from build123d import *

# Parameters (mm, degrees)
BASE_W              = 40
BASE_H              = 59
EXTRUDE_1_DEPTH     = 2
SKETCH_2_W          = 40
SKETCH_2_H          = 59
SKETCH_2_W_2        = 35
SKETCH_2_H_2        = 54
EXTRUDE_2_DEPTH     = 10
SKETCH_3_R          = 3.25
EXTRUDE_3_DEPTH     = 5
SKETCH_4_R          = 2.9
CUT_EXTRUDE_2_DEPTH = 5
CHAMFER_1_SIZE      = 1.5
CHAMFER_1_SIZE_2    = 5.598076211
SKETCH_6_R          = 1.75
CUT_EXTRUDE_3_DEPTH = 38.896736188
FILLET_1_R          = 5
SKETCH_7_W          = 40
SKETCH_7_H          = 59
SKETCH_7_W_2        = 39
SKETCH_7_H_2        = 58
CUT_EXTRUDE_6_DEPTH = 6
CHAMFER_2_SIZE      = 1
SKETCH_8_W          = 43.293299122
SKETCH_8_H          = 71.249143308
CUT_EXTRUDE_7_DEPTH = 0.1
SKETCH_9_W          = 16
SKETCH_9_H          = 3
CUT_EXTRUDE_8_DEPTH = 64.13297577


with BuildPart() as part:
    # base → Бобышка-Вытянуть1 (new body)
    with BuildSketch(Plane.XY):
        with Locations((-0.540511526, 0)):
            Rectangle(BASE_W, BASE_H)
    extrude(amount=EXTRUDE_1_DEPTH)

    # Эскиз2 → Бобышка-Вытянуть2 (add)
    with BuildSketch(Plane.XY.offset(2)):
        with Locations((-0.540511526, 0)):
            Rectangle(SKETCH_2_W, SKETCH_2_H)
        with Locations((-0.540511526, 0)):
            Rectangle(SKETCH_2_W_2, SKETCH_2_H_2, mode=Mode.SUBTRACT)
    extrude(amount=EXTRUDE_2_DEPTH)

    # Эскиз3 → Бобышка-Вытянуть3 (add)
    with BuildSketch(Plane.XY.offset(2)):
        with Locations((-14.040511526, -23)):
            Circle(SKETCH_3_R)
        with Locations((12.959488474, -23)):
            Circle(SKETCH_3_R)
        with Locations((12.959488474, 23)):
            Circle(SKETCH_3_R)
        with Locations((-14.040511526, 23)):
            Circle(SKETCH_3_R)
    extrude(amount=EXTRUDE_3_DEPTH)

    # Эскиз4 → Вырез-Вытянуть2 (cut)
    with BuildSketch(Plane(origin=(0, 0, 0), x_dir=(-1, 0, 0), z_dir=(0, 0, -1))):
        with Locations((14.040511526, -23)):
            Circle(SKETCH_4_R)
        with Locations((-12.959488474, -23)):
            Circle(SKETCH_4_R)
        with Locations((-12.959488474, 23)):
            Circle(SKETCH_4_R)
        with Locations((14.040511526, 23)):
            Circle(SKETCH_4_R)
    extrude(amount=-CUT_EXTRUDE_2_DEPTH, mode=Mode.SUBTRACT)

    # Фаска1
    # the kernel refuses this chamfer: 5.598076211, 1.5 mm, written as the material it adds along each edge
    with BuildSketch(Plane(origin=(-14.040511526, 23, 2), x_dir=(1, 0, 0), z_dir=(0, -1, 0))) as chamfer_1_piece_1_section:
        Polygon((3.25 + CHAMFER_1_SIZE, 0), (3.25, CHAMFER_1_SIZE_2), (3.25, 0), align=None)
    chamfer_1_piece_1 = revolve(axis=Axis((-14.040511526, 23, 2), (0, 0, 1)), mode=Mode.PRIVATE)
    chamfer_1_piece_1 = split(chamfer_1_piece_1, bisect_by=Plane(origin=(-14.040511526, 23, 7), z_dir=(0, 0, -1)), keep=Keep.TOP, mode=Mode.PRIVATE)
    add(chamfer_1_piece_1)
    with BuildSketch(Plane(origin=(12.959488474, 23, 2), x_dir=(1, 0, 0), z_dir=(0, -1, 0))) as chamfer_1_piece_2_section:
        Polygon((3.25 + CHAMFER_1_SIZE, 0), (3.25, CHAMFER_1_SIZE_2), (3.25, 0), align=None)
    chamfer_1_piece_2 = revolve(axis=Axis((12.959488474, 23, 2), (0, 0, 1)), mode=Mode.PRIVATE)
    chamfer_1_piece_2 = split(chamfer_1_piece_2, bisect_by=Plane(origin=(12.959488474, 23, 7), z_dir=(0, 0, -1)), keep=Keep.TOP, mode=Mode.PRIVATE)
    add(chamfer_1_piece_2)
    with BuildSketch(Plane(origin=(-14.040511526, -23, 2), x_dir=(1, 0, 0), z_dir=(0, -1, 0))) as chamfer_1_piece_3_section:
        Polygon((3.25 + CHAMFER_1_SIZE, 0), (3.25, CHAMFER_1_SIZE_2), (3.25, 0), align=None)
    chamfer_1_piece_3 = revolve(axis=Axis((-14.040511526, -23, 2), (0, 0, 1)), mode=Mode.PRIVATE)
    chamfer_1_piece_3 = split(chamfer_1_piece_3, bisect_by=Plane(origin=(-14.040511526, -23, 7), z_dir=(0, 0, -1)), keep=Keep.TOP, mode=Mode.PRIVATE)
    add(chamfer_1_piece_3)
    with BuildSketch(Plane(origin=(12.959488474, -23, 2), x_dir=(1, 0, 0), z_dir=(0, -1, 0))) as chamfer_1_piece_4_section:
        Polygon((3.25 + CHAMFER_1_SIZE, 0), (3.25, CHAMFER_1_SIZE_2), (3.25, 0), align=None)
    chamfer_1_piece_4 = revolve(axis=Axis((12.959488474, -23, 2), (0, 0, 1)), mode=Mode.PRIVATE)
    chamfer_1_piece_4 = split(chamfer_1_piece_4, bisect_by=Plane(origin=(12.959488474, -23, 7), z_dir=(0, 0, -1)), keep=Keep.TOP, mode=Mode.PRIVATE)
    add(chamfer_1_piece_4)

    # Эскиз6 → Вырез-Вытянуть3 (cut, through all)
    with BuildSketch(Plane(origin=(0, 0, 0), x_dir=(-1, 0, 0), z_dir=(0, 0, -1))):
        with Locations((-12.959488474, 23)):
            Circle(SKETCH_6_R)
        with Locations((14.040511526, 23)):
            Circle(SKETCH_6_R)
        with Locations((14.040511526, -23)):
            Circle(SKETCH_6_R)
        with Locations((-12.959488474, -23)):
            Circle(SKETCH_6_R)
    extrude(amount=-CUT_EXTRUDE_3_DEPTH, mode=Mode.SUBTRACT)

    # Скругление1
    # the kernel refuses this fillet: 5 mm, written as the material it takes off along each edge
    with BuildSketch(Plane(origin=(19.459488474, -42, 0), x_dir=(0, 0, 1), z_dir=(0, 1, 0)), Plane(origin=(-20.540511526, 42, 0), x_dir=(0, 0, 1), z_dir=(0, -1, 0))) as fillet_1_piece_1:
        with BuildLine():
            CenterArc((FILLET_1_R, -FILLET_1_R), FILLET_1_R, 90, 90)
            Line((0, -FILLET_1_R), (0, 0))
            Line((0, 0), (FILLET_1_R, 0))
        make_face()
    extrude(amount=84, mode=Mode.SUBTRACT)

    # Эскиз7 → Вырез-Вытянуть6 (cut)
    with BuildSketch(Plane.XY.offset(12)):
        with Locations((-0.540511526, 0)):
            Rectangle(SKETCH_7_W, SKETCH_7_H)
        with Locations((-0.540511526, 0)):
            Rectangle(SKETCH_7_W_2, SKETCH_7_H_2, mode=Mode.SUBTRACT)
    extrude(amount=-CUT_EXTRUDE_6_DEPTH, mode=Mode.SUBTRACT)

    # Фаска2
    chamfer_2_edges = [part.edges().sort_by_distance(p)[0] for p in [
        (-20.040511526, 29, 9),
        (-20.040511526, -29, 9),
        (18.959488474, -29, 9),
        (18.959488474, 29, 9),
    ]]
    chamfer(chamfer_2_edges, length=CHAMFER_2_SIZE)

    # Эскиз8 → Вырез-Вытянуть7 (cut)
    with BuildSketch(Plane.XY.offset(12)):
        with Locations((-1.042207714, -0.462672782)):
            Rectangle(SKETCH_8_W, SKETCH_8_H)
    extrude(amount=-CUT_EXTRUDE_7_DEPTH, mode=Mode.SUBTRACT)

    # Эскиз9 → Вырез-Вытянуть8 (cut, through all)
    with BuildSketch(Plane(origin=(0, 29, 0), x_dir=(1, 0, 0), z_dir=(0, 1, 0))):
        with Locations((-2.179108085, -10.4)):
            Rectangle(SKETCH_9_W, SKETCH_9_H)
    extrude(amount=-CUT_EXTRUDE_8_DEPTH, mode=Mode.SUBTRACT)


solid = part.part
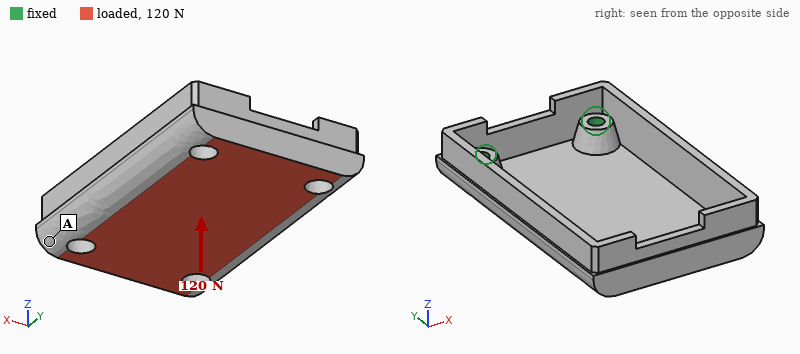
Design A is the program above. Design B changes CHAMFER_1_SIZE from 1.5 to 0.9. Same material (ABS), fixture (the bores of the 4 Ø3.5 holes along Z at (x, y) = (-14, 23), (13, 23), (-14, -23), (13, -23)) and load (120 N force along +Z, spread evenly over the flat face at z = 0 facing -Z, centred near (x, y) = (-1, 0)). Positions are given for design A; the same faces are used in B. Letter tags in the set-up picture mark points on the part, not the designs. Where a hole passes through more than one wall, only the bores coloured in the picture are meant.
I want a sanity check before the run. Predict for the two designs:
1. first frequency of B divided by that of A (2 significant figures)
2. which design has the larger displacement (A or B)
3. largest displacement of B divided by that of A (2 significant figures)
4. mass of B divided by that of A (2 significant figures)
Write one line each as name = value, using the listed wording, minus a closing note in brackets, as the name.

first frequency of B divided by that of A = 0.94
which design has the larger displacement = B
largest displacement of B divided by that of A = 1.1
mass of B divided by that of A = 0.98
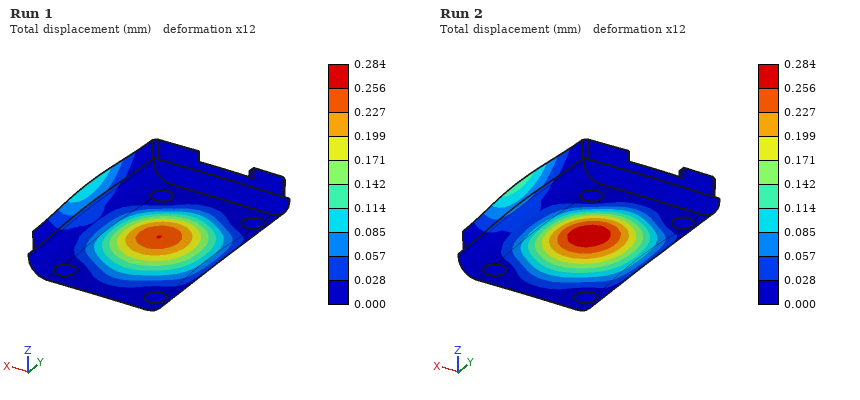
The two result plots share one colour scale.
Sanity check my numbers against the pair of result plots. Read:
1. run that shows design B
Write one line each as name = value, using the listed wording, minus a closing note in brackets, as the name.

run that shows design B = Run 2
